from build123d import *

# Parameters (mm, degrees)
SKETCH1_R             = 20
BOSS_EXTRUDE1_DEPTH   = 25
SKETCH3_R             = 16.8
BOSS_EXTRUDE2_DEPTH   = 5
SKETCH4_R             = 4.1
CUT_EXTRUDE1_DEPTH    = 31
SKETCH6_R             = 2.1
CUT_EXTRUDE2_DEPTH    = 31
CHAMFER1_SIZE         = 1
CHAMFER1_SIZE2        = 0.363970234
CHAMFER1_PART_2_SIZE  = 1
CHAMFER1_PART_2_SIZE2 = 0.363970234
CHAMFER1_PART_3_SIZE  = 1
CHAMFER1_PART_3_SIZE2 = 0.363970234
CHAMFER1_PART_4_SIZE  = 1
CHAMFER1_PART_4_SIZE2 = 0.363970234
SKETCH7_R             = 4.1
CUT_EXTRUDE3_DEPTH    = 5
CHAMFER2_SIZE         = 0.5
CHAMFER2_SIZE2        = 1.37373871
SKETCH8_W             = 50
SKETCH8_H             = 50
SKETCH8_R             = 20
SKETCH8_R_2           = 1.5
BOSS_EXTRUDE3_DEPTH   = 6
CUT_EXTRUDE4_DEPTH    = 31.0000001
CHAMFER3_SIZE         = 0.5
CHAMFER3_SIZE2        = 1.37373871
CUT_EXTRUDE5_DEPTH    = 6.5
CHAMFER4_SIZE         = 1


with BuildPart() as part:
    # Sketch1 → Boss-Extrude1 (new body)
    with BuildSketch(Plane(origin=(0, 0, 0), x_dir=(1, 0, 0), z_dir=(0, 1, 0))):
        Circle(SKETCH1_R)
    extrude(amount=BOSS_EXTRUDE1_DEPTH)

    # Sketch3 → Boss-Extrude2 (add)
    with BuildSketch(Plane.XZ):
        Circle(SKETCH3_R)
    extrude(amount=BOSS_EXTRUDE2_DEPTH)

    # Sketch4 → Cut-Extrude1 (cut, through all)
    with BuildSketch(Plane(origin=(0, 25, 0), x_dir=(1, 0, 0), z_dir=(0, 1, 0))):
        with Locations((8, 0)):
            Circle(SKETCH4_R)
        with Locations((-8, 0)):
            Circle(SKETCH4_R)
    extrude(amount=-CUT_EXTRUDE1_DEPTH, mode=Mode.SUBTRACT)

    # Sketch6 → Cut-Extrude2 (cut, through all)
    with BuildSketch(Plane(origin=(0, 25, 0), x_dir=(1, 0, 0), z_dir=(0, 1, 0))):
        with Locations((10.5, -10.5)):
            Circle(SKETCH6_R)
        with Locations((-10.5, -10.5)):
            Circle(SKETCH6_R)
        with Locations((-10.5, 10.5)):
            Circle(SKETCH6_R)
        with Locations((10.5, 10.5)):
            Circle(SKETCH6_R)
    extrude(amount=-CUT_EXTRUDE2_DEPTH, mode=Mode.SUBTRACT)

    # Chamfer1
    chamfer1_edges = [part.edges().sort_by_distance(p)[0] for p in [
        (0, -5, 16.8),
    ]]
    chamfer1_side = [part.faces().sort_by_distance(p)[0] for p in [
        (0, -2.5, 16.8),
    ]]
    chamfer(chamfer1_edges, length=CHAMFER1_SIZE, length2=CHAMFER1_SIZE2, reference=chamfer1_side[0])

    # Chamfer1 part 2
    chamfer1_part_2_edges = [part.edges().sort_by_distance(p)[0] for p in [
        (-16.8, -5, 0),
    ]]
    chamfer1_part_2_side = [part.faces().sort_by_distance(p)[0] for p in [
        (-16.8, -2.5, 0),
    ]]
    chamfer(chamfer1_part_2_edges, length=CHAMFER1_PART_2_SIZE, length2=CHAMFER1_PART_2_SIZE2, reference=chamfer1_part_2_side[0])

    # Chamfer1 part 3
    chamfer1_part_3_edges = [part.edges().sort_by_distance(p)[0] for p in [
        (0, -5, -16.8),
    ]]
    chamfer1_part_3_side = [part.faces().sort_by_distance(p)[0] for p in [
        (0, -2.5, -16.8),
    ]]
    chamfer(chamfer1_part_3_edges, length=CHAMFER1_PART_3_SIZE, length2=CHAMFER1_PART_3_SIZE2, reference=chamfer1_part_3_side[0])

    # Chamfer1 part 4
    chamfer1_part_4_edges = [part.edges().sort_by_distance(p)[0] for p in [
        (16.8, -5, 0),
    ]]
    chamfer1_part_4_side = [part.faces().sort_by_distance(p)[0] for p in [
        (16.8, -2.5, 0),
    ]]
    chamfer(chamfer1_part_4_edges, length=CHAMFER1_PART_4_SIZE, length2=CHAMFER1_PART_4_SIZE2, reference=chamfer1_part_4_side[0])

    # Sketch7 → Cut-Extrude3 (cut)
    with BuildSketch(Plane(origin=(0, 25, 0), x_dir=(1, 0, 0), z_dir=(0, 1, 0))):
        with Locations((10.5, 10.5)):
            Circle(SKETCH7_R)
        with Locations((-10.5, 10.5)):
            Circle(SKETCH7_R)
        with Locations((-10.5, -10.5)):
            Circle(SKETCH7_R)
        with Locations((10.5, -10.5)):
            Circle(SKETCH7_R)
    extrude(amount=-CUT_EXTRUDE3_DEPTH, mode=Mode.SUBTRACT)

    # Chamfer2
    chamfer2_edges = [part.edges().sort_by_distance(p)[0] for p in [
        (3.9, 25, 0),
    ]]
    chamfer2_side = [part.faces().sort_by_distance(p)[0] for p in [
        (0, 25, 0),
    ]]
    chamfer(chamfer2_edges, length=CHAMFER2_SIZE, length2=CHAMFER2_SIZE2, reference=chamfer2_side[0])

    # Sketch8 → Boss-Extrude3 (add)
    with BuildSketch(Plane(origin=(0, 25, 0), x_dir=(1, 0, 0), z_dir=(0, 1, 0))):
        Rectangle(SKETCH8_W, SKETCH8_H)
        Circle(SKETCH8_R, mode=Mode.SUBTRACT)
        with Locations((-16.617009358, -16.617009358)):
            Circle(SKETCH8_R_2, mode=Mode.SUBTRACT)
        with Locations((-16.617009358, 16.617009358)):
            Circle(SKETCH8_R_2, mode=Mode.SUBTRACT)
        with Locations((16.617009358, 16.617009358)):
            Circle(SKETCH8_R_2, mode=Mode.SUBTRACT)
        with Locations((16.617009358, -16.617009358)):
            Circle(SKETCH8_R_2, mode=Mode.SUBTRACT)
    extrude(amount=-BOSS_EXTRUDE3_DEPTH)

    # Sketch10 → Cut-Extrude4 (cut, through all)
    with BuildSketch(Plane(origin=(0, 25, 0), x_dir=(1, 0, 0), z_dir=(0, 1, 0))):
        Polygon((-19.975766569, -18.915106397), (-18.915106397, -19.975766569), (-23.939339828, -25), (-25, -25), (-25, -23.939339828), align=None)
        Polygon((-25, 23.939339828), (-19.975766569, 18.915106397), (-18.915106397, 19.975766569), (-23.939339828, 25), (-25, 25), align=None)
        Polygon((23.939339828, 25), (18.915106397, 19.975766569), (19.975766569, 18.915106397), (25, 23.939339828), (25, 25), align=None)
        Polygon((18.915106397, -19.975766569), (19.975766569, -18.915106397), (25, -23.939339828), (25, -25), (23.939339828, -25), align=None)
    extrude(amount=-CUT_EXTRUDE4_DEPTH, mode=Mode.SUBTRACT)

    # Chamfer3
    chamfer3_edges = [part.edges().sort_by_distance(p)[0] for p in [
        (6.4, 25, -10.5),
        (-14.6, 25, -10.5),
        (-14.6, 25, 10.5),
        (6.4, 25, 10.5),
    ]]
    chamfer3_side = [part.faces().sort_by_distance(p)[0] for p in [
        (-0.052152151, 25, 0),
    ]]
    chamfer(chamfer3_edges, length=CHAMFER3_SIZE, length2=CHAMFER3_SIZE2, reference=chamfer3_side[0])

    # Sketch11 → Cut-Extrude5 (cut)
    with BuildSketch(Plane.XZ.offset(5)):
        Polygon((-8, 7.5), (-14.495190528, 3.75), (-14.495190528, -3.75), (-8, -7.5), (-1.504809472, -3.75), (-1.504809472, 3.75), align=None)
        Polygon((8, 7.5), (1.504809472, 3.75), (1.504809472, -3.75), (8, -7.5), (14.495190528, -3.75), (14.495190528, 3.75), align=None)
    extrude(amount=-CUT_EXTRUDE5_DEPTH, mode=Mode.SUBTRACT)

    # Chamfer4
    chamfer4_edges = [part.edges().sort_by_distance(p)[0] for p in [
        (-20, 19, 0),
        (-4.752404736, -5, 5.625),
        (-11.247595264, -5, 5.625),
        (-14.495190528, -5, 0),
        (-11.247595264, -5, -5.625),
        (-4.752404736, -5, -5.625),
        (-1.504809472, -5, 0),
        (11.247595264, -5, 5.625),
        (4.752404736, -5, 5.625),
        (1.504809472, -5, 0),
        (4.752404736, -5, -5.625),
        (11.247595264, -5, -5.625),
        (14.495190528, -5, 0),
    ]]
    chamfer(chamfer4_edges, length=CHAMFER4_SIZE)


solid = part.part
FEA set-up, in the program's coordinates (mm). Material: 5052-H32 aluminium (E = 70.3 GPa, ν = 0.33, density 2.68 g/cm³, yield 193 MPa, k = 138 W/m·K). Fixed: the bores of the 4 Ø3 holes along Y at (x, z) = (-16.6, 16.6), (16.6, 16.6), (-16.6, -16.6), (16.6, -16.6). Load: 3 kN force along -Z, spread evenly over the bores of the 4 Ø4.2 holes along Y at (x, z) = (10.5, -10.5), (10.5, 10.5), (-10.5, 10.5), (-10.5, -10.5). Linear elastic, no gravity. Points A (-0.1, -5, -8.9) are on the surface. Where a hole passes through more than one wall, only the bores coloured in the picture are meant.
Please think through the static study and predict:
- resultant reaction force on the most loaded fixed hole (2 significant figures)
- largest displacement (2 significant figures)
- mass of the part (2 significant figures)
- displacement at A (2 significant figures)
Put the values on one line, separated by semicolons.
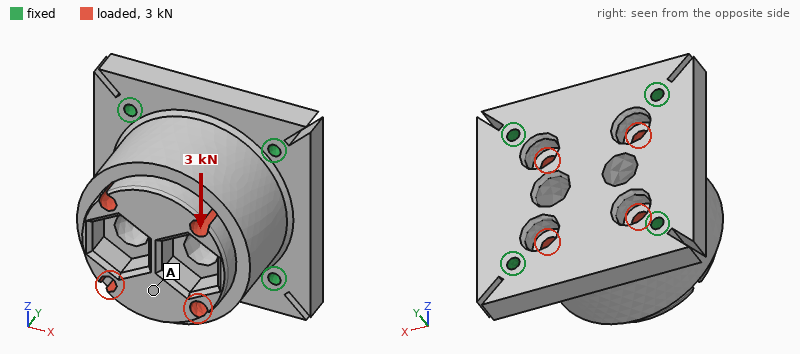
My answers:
1.0 kN; 11 µm; 96 g; 8.6 µm
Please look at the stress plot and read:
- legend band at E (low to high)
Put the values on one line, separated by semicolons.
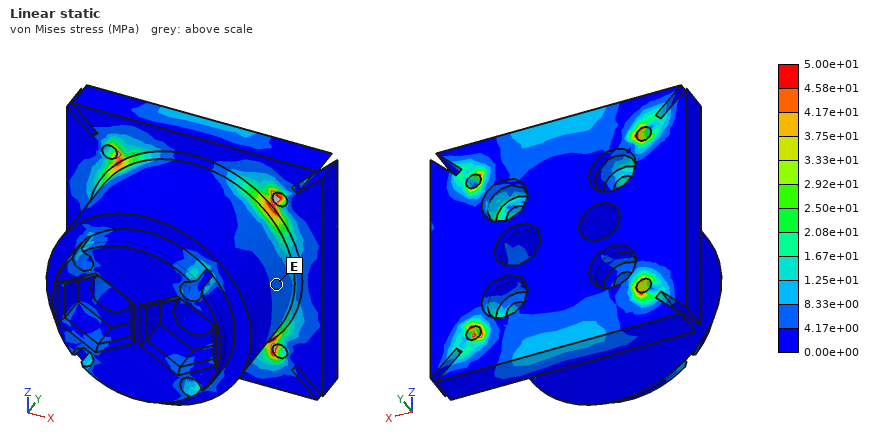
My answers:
4.17e+00 to 8.33e+00 MPa
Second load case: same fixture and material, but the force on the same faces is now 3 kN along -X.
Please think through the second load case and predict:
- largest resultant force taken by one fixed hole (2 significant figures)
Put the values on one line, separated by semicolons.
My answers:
1.0 kN
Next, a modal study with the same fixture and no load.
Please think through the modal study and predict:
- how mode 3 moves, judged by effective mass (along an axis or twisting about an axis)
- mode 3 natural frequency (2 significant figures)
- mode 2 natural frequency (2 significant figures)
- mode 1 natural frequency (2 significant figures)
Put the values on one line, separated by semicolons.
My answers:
along Y; 15 kHz; 13 kHz; 13 kHz
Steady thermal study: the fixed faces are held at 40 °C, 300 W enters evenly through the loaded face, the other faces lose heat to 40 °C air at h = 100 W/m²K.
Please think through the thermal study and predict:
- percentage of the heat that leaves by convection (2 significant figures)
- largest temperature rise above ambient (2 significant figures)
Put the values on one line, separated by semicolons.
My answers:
15 %; 74 K
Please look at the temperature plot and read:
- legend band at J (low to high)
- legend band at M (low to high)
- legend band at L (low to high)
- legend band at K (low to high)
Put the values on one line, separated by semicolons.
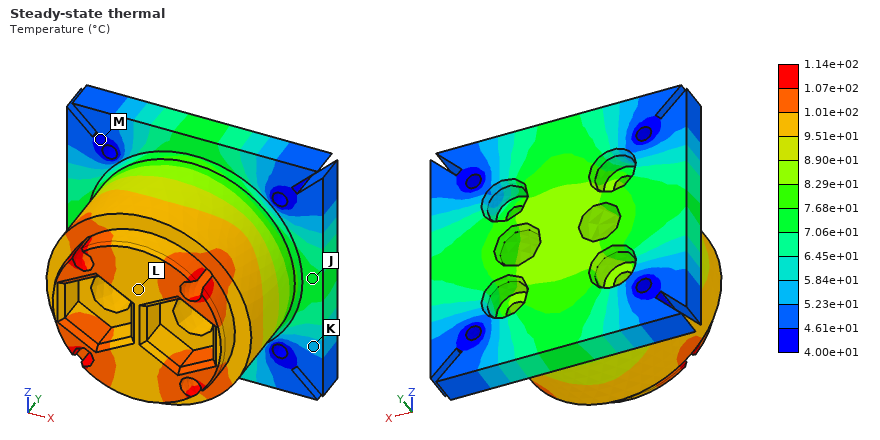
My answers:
7.06e+01 to 7.68e+01 °C; 4.00e+01 to 4.61e+01 °C; 9.51e+01 to 1.01e+02 °C; 5.23e+01 to 5.84e+01 °C
